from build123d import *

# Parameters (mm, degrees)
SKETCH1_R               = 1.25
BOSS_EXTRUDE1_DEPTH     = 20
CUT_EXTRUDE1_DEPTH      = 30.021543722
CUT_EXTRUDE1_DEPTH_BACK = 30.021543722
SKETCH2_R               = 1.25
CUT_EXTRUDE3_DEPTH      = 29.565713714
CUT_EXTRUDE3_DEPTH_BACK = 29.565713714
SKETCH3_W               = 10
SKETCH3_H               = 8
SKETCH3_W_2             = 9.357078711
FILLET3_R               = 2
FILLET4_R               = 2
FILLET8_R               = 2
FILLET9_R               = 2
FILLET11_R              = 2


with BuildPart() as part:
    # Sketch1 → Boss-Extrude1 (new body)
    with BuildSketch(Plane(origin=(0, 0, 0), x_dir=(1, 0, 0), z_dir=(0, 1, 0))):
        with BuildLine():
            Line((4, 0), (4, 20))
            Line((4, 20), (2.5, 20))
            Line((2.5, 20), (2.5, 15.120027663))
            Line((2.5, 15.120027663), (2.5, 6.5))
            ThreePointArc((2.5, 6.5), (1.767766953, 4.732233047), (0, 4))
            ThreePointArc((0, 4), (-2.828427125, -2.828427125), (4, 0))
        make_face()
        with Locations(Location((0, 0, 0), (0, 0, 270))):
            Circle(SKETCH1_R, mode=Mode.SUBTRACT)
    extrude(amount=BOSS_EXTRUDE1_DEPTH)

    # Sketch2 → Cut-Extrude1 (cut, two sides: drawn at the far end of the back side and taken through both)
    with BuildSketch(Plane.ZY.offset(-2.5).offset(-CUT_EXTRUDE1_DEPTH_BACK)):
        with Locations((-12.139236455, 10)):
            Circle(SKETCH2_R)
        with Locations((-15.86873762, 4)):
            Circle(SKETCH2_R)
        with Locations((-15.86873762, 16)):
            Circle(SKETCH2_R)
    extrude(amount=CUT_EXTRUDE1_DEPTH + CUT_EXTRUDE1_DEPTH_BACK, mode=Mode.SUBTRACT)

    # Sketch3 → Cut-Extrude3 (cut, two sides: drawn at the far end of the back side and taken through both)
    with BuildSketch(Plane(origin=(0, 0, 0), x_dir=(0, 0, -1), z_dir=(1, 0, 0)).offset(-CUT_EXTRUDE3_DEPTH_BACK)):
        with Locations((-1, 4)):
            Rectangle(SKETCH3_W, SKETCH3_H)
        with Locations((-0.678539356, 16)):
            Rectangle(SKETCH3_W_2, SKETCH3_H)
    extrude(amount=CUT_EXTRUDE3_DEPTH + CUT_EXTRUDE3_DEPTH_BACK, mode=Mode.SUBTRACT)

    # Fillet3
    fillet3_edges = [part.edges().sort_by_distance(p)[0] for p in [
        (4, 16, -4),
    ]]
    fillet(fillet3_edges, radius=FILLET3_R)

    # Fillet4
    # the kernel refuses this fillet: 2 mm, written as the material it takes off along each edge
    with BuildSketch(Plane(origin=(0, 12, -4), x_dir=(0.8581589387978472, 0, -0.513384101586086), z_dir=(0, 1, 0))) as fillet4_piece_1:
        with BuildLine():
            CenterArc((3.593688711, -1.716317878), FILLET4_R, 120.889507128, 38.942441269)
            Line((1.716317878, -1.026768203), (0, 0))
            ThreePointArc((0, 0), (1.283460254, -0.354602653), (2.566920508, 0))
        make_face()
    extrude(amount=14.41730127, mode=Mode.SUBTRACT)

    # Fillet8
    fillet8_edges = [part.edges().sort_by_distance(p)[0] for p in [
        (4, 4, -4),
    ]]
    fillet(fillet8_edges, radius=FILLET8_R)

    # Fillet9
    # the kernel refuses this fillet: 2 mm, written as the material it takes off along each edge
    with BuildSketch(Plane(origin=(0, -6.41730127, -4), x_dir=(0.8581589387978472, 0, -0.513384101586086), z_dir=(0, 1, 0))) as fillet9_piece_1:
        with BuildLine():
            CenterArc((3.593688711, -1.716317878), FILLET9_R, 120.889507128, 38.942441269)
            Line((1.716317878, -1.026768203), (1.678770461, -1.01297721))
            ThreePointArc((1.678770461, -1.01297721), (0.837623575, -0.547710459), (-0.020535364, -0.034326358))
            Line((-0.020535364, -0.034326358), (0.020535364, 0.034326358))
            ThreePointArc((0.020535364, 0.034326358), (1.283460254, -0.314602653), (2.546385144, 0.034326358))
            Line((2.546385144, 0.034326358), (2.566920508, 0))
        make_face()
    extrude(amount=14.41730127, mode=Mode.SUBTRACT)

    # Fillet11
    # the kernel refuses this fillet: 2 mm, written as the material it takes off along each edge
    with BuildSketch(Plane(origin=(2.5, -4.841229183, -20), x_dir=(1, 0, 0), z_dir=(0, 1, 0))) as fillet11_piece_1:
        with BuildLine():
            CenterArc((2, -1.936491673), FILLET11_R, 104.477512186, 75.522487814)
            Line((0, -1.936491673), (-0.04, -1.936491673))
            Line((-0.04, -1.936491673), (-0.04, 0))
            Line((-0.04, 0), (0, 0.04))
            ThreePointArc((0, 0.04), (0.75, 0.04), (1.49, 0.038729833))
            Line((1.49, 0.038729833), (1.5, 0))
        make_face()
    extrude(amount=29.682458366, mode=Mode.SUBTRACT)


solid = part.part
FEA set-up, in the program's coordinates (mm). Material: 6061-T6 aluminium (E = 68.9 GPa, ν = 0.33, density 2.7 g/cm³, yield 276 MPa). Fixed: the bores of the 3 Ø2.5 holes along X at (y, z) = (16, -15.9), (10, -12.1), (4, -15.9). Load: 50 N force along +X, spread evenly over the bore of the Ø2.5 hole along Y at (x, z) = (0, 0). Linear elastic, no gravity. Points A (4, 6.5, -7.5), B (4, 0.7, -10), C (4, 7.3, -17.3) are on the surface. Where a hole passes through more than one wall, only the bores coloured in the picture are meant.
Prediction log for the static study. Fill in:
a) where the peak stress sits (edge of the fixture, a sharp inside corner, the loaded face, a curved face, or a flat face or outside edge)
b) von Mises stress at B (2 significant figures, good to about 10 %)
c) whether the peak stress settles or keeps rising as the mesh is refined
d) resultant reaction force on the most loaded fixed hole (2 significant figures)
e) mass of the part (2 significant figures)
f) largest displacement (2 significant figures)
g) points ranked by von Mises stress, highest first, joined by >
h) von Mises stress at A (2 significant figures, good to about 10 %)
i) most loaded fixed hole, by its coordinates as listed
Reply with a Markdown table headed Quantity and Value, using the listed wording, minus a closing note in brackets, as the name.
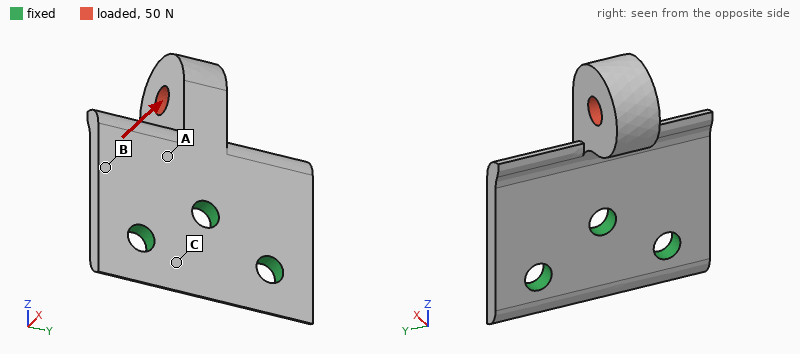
| Quantity | Value |
|---|---|
| where the peak stress sits | edge of the fixture |
| von Mises stress at B | 36 MPa |
| whether the peak stress settles or keeps rising as the mesh is refined | keeps rising |
| resultant reaction force on the most loaded fixed hole | 85 N |
| mass of the part | 1.7 g |
| largest displacement | 0.16 mm |
| points ranked by von Mises stress, highest first, joined by > | A > B > C |
| von Mises stress at A | 62 MPa |
| most loaded fixed hole, by its coordinates as listed | (10, -12.1) |
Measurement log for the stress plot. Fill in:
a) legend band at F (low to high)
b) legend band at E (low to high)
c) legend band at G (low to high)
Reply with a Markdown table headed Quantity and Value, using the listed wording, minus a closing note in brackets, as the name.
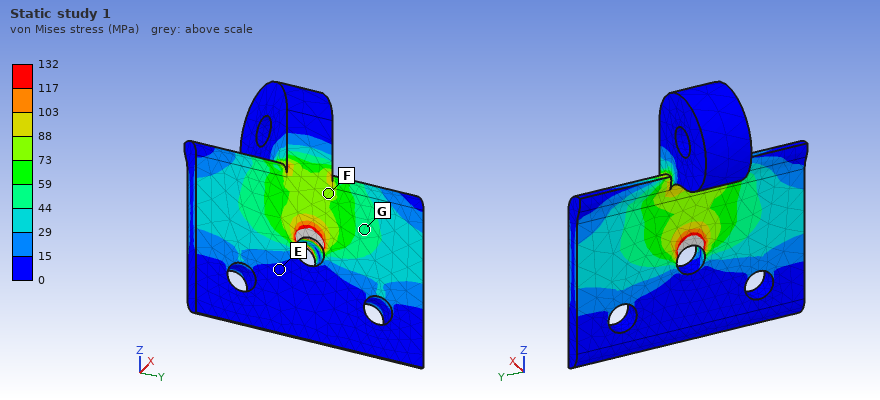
| Quantity | Value |
|---|---|
| legend band at F | 73 to 88 MPa |
| legend band at E | 0 to 15 MPa |
| legend band at G | 44 to 59 MPa |
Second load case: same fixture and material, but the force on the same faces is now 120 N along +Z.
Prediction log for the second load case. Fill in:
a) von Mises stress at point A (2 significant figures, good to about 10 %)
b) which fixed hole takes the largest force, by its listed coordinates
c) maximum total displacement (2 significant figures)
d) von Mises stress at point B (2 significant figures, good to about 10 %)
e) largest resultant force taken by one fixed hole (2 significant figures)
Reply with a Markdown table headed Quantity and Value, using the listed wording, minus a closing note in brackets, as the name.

| Quantity | Value |
|---|---|
| von Mises stress at point A | 56 MPa |
| which fixed hole takes the largest force, by its listed coordinates | (10, -12.1) |
| maximum total displacement | 0.16 mm |
| von Mises stress at point B | 30 MPa |
| largest resultant force taken by one fixed hole | 81 N |
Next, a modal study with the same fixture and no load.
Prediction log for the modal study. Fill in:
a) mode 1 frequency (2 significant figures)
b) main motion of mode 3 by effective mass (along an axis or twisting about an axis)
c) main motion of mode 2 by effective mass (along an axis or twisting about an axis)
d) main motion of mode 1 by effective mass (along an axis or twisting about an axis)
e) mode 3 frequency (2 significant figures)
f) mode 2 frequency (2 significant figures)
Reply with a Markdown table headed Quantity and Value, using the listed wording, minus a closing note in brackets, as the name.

| Quantity | Value |
|---|---|
| mode 1 frequency | 4300 Hz |
| main motion of mode 3 by effective mass | along X |
| main motion of mode 2 by effective mass | along Y |
| main motion of mode 1 by effective mass | along X |
| mode 3 frequency | 18 kHz |
| mode 2 frequency | 11 kHz |
